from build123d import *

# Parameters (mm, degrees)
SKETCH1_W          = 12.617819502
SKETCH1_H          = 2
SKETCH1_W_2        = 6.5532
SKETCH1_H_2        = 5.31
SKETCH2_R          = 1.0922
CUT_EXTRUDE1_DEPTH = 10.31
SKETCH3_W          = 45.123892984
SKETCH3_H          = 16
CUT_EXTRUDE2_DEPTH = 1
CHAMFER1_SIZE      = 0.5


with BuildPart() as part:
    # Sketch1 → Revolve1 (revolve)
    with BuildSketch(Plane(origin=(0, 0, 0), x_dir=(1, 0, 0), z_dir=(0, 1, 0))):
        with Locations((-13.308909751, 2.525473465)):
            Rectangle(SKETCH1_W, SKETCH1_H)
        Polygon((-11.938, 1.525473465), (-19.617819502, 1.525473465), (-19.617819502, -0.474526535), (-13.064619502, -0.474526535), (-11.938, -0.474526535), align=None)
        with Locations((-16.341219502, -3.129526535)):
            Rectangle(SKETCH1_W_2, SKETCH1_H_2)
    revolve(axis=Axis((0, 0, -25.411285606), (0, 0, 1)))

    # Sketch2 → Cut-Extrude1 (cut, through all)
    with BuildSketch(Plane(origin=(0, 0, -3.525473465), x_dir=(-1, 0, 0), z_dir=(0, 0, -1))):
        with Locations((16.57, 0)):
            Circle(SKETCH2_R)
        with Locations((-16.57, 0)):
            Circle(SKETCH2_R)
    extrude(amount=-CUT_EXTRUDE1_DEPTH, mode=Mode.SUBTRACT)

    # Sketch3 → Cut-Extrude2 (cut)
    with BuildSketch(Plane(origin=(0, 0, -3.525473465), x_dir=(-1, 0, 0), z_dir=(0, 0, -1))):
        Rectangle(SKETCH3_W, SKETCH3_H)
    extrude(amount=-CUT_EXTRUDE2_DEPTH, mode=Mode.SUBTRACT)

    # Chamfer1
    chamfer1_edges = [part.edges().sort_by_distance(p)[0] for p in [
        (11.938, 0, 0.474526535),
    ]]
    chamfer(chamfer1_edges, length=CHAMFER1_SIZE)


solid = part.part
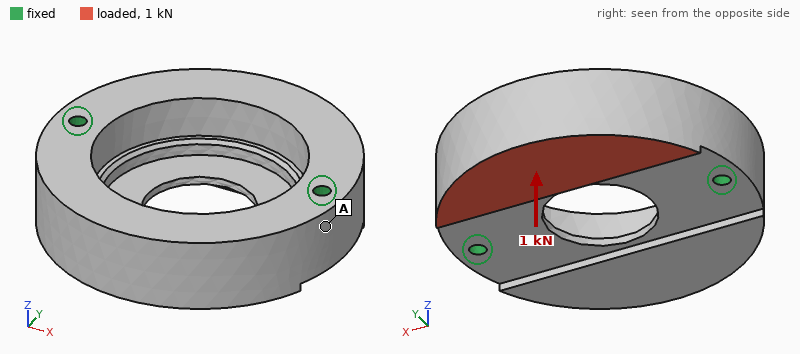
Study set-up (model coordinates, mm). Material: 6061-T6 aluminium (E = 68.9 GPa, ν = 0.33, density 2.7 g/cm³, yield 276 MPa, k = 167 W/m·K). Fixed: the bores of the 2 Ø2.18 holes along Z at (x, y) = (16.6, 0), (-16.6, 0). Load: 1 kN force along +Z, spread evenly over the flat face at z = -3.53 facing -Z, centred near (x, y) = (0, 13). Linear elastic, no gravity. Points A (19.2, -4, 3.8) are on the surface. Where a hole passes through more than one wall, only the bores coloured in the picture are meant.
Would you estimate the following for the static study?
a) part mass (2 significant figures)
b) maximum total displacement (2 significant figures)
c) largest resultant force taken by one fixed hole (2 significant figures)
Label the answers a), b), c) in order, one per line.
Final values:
a) 18 g
b) 43 µm
c) 530 N
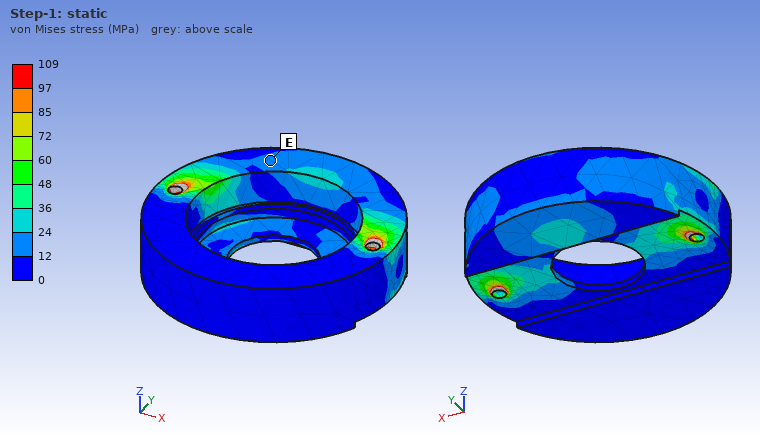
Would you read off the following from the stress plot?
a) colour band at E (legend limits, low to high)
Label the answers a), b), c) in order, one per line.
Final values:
a) 12 to 24 MPa
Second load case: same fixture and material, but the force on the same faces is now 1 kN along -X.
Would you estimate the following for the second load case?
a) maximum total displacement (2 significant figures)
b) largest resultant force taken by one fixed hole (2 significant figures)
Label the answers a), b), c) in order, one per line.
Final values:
a) 9.6 µm
b) 610 N
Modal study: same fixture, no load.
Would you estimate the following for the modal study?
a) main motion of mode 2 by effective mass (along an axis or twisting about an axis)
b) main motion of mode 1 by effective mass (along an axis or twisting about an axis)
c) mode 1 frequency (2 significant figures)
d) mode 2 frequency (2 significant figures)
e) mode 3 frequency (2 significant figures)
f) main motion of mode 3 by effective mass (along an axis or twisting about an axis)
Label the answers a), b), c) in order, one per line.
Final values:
a) along Z
b) twisting about X
c) 11 kHz
d) 12 kHz
e) 20 kHz
f) twisting about Z
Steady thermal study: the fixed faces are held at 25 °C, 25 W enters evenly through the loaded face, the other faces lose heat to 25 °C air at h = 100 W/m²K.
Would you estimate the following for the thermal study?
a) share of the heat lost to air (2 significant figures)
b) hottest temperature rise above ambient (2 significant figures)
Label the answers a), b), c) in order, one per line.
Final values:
a) 7.9 %
b) 19 K
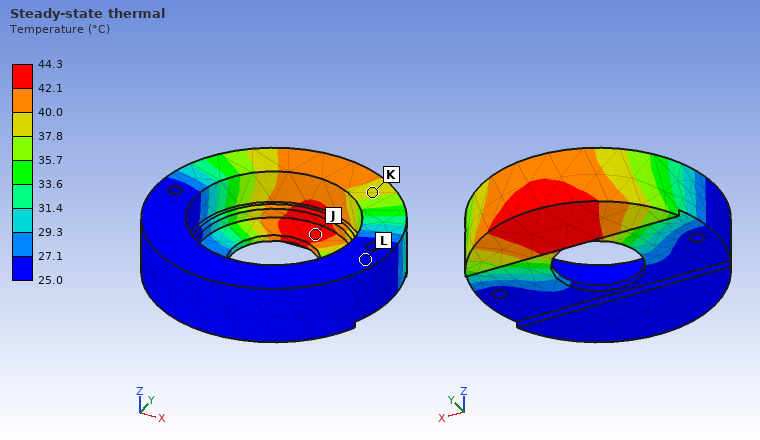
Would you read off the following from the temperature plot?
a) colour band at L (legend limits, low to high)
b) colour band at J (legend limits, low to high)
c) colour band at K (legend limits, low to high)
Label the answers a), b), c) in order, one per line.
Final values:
a) 25.0 to 27.1 °C
b) 42.1 to 44.3 °C
c) 37.8 to 40.0 °C
